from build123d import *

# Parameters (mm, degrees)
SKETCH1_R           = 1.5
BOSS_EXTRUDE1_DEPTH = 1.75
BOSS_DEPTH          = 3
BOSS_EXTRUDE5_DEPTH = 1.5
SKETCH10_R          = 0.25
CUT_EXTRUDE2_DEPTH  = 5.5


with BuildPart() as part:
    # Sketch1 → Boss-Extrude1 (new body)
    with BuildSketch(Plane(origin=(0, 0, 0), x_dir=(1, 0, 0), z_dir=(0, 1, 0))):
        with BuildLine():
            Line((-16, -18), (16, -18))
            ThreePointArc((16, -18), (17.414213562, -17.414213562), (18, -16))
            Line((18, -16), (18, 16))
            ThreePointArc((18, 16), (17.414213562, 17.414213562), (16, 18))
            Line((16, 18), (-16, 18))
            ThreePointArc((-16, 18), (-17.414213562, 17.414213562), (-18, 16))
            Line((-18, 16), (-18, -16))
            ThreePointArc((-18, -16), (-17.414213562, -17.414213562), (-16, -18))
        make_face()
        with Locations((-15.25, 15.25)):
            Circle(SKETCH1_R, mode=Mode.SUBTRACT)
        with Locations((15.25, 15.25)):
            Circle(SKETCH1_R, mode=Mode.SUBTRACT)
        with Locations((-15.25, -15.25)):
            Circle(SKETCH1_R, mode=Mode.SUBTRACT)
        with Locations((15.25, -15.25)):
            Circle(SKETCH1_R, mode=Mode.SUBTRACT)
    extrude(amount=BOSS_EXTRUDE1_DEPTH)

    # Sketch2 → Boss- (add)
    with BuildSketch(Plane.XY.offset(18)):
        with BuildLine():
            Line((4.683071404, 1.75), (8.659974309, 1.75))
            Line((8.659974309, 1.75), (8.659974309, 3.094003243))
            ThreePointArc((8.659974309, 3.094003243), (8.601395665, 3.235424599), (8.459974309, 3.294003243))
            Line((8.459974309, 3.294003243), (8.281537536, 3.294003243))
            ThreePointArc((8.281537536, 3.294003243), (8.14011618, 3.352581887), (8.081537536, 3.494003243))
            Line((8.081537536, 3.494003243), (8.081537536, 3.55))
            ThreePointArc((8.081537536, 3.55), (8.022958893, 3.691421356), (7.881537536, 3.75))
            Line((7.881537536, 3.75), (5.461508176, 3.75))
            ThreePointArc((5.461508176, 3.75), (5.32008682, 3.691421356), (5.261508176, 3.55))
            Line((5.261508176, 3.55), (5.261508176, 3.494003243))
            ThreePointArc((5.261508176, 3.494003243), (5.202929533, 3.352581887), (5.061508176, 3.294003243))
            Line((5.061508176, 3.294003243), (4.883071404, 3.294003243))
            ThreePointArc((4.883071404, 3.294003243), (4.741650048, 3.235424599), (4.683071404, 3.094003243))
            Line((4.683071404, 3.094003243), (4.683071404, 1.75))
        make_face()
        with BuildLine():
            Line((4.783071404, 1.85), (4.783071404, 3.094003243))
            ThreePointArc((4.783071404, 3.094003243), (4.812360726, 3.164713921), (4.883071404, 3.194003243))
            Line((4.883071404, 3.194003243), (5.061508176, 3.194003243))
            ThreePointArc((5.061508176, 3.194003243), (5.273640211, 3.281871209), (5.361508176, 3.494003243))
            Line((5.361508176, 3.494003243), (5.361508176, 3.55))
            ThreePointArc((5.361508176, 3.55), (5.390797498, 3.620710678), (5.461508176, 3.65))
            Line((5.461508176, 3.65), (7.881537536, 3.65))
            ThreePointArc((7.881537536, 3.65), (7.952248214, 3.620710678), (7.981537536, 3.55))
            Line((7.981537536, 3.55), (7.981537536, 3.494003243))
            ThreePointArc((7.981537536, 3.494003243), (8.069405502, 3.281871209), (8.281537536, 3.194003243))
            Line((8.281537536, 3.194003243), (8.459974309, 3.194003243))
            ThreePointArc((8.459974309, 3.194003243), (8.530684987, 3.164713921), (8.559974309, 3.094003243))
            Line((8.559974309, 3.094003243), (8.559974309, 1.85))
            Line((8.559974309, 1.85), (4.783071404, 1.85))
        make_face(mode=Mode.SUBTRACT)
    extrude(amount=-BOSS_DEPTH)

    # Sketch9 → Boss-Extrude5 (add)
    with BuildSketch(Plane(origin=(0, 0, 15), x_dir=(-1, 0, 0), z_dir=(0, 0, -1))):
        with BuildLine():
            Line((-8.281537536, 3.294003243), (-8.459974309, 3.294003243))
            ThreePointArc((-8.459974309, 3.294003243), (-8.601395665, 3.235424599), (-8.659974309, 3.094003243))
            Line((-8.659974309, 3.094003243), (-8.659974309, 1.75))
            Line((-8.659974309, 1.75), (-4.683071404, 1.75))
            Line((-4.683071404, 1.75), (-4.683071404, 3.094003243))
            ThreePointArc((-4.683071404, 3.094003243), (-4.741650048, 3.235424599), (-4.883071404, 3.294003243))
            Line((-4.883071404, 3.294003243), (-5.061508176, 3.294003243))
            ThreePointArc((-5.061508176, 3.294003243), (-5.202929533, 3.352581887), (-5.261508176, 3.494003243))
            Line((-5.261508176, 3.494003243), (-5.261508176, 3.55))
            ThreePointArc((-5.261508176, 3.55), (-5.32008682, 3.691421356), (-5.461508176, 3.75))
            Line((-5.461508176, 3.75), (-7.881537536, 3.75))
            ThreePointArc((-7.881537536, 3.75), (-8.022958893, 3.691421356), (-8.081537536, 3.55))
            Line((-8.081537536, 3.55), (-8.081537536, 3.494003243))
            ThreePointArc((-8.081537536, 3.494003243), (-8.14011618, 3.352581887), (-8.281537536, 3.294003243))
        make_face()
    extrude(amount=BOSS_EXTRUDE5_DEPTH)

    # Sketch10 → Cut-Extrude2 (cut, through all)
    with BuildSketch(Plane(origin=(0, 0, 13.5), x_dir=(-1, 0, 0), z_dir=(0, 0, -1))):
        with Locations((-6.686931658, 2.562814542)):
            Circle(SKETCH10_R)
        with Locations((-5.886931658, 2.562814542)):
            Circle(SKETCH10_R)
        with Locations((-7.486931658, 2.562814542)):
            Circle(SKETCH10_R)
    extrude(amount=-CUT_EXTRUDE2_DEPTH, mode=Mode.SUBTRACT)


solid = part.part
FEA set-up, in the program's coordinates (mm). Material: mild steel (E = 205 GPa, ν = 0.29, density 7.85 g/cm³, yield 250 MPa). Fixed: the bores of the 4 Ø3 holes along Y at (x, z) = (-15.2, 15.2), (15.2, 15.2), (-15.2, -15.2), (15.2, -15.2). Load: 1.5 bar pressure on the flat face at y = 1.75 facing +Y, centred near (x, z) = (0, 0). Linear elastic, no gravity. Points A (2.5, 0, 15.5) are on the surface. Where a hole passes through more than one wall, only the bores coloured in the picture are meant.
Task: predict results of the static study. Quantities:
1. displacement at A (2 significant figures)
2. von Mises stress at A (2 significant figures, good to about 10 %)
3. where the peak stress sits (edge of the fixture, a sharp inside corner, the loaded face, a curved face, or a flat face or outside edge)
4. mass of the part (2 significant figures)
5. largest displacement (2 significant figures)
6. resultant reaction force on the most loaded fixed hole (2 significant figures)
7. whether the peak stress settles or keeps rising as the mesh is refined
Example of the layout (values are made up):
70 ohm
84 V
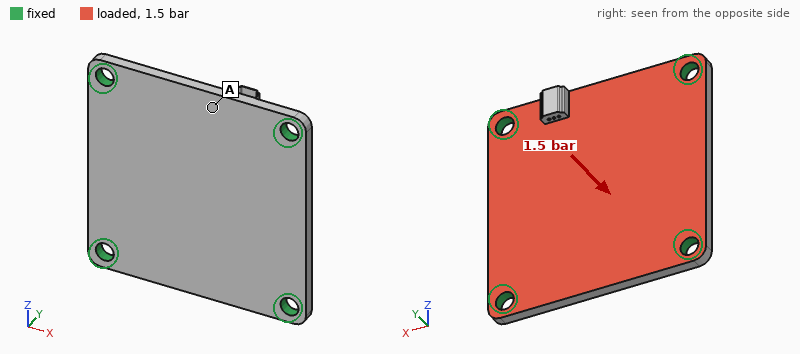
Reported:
3.8 µm
12 MPa
edge of the fixture
17 g
8.4 µm
47 N
keeps rising
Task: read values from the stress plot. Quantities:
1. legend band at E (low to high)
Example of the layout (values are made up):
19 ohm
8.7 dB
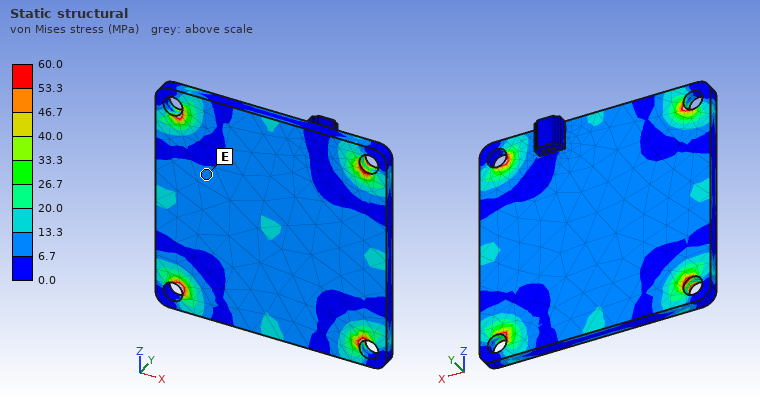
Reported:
6.7 to 13.3 MPa
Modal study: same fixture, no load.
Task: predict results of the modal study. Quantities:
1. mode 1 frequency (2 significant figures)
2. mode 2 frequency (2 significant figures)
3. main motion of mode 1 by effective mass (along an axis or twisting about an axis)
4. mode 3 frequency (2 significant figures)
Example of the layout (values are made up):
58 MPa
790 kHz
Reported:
7000 Hz
12 kHz
along Y
12 kHz
